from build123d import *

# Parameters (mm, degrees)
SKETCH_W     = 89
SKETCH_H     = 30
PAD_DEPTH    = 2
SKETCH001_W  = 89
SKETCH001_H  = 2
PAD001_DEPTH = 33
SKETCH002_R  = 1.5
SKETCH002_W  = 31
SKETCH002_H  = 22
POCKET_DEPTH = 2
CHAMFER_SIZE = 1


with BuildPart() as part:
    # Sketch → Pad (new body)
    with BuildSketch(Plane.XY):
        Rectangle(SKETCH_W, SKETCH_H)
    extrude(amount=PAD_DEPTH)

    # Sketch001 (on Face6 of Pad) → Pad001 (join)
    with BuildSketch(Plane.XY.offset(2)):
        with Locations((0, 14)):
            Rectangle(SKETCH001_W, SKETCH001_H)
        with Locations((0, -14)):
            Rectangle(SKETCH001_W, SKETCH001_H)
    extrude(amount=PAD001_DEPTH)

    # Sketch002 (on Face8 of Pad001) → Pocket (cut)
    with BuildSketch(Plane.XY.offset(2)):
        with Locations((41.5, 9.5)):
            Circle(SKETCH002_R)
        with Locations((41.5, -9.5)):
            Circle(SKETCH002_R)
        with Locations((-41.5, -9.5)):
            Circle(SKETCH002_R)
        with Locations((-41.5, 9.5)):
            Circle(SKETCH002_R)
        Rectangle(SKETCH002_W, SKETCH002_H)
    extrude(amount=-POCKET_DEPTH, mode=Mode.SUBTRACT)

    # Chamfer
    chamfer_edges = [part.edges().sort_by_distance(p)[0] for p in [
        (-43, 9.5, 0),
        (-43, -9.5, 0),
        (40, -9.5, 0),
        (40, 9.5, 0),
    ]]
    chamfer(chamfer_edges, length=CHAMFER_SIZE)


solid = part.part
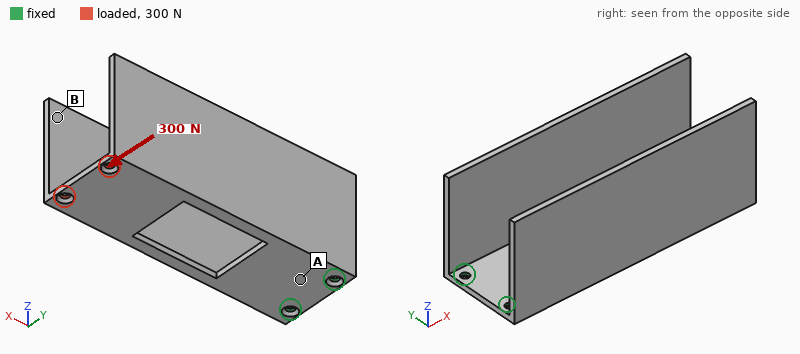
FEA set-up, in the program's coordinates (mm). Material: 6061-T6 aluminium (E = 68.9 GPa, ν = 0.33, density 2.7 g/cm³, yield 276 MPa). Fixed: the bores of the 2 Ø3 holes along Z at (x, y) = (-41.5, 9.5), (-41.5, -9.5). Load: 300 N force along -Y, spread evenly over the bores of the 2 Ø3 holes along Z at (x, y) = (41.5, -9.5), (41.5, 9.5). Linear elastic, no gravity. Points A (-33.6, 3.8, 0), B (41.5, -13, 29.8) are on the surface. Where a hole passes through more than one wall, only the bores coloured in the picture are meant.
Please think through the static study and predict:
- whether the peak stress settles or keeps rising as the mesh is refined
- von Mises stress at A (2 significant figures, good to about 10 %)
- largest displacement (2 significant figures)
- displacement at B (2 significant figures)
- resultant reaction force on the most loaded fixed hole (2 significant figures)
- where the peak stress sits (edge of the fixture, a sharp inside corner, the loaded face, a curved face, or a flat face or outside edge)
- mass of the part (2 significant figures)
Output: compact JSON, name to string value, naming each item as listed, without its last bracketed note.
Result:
{"whether the peak stress settles or keeps rising as the mesh is refined": "keeps rising", "von Mises stress at A": "34 MPa", "largest displacement": "0.66 mm", "displacement at B": "0.63 mm", "resultant reaction force on the most loaded fixed hole": "1.2 kN", "where the peak stress sits": "edge of the fixture", "mass of the part": "42 g"}
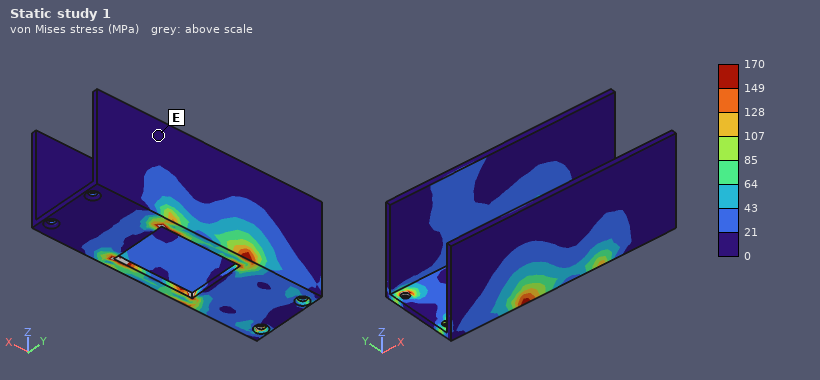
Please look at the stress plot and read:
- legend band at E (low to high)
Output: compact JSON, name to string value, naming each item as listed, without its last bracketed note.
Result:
{"legend band at E": "0 to 21 MPa"}
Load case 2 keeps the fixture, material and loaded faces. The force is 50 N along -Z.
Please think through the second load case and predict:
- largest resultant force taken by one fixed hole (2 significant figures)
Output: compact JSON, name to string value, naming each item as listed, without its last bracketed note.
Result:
{"largest resultant force taken by one fixed hole": "36 N"}
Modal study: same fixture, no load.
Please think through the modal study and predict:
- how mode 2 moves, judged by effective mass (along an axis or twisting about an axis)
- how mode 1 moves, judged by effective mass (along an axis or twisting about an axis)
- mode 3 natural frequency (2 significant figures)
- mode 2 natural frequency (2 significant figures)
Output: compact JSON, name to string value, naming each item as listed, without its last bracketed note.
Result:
{"how mode 2 moves, judged by effective mass": "along Y", "how mode 1 moves, judged by effective mass": "along Z", "mode 3 natural frequency": "790 Hz", "mode 2 natural frequency": "410 Hz"}
